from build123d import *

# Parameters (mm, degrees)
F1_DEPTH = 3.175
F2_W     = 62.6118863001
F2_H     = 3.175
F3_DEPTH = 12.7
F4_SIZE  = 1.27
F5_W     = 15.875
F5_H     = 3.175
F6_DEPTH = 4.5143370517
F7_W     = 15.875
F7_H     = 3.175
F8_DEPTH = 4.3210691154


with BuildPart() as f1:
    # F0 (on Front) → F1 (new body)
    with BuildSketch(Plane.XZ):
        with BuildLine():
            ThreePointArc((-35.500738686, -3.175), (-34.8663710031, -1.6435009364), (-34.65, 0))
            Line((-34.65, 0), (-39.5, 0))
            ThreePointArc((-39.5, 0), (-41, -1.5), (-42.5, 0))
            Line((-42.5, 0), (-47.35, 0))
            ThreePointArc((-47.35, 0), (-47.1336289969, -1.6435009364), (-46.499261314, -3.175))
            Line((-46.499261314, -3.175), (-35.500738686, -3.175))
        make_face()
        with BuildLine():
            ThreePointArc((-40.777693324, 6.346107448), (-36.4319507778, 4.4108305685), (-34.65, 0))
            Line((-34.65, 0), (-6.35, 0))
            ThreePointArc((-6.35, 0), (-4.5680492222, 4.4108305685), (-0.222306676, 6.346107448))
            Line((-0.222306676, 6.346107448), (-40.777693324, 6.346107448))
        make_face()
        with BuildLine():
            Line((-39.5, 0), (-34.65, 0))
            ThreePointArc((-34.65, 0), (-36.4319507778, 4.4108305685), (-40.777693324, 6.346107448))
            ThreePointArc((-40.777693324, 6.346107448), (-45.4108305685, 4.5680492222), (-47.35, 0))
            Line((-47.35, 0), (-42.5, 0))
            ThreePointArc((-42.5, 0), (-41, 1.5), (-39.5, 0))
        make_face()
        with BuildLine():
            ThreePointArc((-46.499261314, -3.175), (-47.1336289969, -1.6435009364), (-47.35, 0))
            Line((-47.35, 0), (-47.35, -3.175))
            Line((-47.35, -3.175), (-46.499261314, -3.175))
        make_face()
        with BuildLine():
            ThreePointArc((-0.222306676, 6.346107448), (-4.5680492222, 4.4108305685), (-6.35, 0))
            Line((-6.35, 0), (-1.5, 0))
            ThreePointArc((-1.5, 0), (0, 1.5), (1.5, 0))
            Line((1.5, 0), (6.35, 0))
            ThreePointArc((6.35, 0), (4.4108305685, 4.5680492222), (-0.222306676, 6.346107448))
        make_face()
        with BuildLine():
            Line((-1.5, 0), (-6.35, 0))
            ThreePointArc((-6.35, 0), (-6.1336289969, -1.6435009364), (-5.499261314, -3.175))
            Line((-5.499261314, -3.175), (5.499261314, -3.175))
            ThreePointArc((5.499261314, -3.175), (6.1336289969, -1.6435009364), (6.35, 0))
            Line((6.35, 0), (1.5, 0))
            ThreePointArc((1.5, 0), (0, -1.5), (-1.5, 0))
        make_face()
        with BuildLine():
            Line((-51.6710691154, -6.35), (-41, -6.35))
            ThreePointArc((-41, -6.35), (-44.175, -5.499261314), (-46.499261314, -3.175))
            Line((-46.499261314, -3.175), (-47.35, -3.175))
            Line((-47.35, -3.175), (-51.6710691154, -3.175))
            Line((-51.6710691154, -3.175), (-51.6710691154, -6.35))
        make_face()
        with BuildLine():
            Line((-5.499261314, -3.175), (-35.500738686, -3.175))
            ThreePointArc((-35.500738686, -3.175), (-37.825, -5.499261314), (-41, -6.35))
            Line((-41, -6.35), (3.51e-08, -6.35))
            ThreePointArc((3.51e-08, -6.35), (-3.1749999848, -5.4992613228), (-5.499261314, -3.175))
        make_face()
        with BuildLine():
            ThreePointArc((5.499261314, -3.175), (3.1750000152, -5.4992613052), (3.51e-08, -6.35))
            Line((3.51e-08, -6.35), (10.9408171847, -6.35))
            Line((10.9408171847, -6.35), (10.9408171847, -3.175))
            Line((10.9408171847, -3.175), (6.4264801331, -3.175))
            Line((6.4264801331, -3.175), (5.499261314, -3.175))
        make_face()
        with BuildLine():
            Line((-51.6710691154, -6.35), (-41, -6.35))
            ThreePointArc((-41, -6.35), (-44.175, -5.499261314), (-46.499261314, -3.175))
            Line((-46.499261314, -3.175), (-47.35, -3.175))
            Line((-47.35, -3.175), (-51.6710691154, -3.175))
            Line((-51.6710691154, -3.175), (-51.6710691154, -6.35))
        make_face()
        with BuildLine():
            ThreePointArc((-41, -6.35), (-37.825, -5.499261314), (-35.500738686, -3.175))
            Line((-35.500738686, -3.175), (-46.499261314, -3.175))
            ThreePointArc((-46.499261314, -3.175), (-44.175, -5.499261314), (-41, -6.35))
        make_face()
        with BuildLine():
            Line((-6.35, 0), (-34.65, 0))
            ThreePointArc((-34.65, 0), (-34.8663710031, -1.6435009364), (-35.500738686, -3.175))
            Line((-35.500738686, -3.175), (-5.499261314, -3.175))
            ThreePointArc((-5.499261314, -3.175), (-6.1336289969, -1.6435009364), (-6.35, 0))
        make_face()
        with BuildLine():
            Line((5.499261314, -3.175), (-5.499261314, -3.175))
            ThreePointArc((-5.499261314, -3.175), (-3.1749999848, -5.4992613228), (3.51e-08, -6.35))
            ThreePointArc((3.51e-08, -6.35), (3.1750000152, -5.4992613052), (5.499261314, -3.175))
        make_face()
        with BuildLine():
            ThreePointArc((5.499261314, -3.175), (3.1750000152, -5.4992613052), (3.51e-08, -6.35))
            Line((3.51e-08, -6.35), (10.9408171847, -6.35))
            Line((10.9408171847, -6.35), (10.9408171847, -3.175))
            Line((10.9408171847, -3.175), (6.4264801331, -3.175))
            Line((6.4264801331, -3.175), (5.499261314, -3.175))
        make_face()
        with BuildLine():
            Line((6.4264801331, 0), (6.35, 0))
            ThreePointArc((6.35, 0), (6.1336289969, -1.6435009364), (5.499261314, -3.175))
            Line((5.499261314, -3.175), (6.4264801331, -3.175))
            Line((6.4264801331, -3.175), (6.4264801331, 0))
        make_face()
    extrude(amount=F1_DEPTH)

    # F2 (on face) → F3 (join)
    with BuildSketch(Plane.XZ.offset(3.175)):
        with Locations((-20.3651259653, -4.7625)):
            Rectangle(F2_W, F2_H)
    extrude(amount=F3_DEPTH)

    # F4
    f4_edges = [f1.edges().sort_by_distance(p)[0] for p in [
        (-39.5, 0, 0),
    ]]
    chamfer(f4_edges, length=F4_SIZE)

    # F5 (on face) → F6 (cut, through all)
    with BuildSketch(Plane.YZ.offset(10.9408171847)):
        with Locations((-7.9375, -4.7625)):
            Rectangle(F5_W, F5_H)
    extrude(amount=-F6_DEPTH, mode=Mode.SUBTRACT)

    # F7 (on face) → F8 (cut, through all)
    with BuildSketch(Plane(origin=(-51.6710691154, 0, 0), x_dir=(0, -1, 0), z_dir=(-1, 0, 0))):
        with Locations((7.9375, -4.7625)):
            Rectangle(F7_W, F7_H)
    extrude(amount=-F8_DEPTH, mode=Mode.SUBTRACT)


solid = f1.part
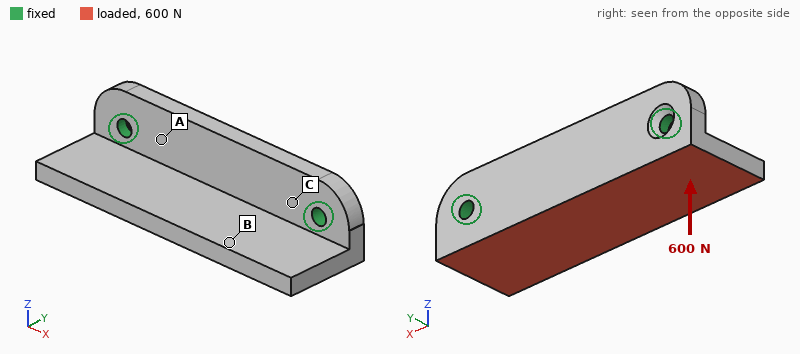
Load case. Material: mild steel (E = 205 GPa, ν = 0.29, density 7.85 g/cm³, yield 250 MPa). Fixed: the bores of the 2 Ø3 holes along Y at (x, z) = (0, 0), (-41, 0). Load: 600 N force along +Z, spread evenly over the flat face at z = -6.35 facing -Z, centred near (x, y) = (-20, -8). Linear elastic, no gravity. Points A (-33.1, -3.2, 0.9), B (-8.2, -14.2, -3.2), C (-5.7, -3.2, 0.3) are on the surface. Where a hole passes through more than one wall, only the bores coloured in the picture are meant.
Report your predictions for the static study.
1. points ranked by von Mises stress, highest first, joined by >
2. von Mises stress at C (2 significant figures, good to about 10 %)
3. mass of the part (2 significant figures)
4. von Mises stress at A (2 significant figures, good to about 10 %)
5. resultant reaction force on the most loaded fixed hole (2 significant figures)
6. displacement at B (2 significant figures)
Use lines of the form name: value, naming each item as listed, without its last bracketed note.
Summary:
points ranked by von Mises stress, highest first, joined by >: C > A > B
von Mises stress at C: 44 MPa
mass of the part: 33 g
von Mises stress at A: 33 MPa
resultant reaction force on the most loaded fixed hole: 300 N
displacement at B: 20 µm
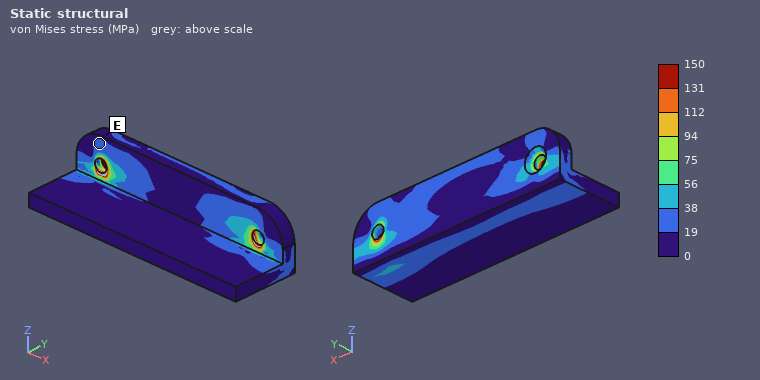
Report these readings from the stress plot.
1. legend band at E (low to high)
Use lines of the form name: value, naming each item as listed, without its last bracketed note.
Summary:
legend band at E: 19 to 38 MPa
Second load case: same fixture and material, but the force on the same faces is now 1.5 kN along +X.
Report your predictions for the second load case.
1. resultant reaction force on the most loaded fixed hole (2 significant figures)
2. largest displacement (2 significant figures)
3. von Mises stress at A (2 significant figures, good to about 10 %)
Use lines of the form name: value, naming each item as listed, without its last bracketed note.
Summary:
resultant reaction force on the most loaded fixed hole: 830 N
largest displacement: 4.0 µm
von Mises stress at A: 17 MPa
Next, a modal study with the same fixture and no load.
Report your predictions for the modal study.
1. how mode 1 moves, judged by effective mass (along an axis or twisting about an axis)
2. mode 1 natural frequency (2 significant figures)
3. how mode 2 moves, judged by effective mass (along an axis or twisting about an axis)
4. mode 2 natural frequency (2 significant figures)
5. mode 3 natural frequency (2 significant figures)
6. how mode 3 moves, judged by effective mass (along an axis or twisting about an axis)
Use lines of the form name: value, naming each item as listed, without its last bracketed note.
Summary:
how mode 1 moves, judged by effective mass: along Z
mode 1 natural frequency: 6200 Hz
how mode 2 moves, judged by effective mass: twisting about Y
mode 2 natural frequency: 10 kHz
mode 3 natural frequency: 14 kHz
how mode 3 moves, judged by effective mass: along Y
